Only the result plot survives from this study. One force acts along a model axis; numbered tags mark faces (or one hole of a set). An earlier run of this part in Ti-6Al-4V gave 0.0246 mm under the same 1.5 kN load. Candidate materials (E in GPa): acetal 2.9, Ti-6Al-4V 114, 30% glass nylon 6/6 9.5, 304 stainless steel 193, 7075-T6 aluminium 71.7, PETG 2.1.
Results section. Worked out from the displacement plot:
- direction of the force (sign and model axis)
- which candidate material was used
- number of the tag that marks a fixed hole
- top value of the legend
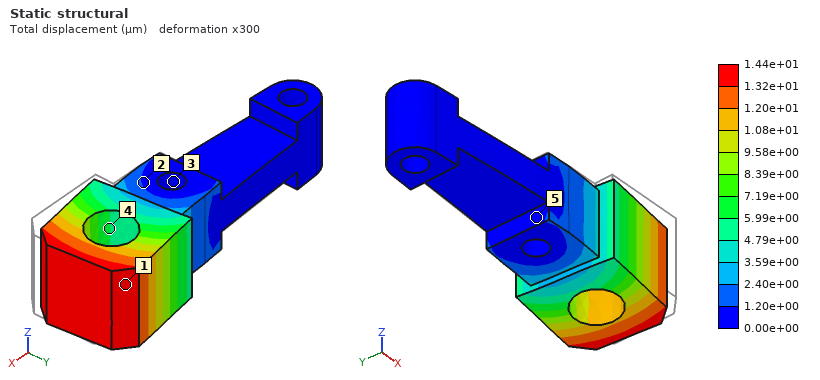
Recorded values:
+Y
304 stainless steel
3
1.44e+01 µm
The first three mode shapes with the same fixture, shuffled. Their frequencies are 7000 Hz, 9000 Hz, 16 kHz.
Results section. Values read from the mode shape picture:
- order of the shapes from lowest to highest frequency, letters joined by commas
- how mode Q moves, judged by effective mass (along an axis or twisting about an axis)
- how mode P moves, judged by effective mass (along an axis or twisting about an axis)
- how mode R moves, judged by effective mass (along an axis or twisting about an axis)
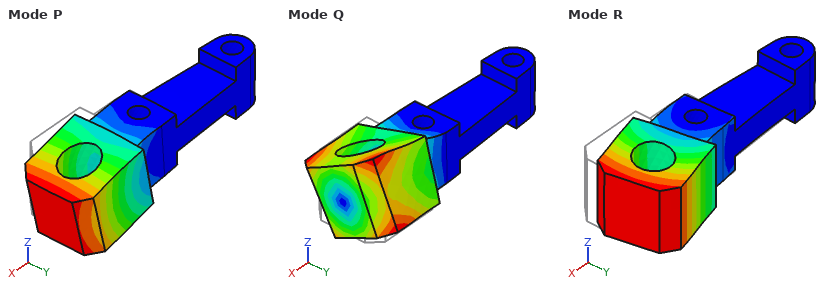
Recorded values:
R, P, Q
twisting about X
along Z
along Y
